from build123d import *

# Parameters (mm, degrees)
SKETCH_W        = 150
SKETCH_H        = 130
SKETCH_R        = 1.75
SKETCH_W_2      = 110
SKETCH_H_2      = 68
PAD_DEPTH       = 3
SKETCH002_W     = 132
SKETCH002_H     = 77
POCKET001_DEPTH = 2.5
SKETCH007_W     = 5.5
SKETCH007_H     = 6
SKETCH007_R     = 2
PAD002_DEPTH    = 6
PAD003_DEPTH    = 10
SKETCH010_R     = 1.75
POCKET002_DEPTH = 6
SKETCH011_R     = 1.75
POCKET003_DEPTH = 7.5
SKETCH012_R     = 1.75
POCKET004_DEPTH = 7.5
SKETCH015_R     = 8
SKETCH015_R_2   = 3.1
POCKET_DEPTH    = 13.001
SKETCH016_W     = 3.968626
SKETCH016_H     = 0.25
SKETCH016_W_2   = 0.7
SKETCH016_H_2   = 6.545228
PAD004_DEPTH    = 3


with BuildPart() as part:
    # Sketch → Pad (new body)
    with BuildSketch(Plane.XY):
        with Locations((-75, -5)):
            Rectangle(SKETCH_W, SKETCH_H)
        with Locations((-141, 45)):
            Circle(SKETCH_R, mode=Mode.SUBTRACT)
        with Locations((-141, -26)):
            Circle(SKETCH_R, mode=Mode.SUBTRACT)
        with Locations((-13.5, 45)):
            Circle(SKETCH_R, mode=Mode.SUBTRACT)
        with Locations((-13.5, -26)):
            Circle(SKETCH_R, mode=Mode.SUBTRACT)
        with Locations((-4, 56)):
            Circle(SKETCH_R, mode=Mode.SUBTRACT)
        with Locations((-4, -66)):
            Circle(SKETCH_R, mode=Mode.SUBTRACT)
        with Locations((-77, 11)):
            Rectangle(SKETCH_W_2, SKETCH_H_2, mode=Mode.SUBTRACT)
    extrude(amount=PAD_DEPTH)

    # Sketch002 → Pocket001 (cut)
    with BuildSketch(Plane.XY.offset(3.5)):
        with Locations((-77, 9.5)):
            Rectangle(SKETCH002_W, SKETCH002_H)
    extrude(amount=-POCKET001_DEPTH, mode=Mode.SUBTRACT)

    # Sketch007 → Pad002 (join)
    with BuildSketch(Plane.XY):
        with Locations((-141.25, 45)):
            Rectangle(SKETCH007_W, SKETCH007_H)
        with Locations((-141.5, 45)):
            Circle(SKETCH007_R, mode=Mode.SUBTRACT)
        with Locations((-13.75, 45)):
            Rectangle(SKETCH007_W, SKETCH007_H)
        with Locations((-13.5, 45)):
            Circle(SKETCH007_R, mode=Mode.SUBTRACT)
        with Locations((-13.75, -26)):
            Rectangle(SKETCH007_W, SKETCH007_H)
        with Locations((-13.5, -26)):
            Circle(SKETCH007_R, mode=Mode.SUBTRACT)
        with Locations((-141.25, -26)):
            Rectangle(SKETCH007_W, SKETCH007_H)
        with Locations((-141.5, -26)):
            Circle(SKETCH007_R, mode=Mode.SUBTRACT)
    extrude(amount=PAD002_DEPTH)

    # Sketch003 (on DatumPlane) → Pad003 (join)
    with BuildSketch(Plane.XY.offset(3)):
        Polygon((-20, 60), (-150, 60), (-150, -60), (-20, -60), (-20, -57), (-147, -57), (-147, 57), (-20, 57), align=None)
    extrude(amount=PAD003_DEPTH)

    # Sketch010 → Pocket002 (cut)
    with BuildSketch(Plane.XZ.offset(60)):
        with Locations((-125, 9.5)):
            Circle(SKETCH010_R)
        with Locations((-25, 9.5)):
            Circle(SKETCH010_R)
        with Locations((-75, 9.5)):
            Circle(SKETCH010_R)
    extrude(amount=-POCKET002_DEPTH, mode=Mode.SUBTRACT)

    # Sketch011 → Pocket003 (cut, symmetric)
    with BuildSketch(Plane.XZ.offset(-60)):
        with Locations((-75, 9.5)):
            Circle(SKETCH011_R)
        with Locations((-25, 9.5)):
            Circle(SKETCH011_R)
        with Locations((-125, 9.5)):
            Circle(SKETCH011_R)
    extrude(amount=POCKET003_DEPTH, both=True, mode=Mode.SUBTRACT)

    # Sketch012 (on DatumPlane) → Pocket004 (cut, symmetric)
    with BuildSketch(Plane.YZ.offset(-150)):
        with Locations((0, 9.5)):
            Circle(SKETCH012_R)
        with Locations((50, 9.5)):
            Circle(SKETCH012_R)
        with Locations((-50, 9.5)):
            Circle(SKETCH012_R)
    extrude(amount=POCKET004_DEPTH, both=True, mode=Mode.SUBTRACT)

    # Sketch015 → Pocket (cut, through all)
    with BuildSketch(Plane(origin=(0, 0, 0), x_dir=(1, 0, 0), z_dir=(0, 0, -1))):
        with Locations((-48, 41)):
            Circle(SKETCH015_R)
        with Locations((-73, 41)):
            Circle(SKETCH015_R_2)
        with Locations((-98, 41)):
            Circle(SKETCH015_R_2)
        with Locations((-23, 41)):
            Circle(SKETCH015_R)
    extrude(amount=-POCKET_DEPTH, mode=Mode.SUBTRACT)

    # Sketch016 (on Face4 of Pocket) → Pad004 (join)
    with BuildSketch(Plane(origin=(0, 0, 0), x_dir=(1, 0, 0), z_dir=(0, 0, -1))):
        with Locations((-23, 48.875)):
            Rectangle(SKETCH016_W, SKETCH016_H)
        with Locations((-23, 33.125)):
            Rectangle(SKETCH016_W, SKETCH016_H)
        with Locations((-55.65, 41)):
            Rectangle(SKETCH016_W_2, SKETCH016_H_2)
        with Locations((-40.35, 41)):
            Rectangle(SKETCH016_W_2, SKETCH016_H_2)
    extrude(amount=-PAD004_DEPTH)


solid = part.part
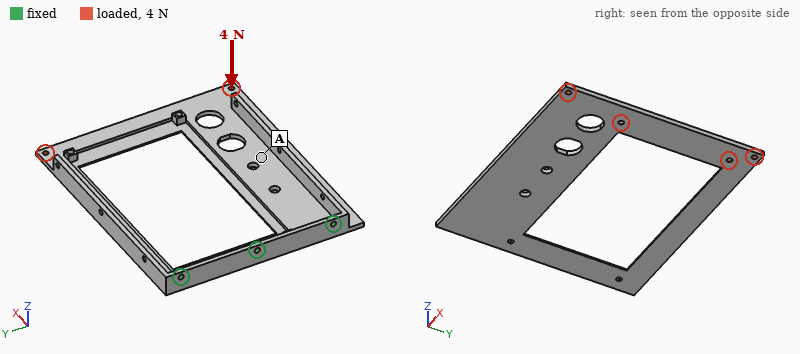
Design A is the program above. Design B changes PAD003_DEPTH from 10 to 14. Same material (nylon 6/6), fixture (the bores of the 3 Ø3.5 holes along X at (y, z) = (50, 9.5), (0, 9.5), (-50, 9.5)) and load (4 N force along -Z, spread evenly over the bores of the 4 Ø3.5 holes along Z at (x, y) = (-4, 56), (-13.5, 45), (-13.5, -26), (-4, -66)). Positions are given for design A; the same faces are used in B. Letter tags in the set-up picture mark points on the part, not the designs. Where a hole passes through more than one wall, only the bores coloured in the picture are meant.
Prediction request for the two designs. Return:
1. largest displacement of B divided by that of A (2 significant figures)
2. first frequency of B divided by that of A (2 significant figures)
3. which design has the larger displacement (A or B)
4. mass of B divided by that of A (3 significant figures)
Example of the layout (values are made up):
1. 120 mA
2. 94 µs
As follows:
1. 0.65
2. 1.2
3. A
4. 1.11
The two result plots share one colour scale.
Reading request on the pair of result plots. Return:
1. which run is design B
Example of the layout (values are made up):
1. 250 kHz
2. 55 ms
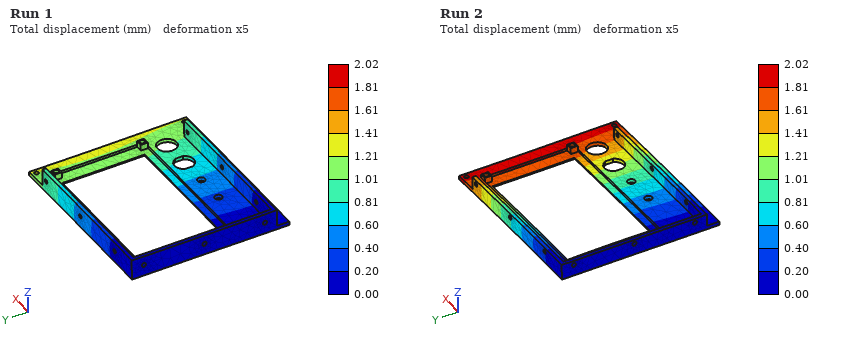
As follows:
1. Run 1
